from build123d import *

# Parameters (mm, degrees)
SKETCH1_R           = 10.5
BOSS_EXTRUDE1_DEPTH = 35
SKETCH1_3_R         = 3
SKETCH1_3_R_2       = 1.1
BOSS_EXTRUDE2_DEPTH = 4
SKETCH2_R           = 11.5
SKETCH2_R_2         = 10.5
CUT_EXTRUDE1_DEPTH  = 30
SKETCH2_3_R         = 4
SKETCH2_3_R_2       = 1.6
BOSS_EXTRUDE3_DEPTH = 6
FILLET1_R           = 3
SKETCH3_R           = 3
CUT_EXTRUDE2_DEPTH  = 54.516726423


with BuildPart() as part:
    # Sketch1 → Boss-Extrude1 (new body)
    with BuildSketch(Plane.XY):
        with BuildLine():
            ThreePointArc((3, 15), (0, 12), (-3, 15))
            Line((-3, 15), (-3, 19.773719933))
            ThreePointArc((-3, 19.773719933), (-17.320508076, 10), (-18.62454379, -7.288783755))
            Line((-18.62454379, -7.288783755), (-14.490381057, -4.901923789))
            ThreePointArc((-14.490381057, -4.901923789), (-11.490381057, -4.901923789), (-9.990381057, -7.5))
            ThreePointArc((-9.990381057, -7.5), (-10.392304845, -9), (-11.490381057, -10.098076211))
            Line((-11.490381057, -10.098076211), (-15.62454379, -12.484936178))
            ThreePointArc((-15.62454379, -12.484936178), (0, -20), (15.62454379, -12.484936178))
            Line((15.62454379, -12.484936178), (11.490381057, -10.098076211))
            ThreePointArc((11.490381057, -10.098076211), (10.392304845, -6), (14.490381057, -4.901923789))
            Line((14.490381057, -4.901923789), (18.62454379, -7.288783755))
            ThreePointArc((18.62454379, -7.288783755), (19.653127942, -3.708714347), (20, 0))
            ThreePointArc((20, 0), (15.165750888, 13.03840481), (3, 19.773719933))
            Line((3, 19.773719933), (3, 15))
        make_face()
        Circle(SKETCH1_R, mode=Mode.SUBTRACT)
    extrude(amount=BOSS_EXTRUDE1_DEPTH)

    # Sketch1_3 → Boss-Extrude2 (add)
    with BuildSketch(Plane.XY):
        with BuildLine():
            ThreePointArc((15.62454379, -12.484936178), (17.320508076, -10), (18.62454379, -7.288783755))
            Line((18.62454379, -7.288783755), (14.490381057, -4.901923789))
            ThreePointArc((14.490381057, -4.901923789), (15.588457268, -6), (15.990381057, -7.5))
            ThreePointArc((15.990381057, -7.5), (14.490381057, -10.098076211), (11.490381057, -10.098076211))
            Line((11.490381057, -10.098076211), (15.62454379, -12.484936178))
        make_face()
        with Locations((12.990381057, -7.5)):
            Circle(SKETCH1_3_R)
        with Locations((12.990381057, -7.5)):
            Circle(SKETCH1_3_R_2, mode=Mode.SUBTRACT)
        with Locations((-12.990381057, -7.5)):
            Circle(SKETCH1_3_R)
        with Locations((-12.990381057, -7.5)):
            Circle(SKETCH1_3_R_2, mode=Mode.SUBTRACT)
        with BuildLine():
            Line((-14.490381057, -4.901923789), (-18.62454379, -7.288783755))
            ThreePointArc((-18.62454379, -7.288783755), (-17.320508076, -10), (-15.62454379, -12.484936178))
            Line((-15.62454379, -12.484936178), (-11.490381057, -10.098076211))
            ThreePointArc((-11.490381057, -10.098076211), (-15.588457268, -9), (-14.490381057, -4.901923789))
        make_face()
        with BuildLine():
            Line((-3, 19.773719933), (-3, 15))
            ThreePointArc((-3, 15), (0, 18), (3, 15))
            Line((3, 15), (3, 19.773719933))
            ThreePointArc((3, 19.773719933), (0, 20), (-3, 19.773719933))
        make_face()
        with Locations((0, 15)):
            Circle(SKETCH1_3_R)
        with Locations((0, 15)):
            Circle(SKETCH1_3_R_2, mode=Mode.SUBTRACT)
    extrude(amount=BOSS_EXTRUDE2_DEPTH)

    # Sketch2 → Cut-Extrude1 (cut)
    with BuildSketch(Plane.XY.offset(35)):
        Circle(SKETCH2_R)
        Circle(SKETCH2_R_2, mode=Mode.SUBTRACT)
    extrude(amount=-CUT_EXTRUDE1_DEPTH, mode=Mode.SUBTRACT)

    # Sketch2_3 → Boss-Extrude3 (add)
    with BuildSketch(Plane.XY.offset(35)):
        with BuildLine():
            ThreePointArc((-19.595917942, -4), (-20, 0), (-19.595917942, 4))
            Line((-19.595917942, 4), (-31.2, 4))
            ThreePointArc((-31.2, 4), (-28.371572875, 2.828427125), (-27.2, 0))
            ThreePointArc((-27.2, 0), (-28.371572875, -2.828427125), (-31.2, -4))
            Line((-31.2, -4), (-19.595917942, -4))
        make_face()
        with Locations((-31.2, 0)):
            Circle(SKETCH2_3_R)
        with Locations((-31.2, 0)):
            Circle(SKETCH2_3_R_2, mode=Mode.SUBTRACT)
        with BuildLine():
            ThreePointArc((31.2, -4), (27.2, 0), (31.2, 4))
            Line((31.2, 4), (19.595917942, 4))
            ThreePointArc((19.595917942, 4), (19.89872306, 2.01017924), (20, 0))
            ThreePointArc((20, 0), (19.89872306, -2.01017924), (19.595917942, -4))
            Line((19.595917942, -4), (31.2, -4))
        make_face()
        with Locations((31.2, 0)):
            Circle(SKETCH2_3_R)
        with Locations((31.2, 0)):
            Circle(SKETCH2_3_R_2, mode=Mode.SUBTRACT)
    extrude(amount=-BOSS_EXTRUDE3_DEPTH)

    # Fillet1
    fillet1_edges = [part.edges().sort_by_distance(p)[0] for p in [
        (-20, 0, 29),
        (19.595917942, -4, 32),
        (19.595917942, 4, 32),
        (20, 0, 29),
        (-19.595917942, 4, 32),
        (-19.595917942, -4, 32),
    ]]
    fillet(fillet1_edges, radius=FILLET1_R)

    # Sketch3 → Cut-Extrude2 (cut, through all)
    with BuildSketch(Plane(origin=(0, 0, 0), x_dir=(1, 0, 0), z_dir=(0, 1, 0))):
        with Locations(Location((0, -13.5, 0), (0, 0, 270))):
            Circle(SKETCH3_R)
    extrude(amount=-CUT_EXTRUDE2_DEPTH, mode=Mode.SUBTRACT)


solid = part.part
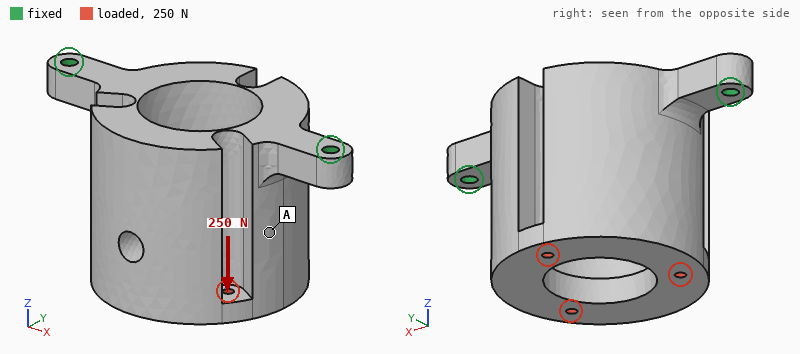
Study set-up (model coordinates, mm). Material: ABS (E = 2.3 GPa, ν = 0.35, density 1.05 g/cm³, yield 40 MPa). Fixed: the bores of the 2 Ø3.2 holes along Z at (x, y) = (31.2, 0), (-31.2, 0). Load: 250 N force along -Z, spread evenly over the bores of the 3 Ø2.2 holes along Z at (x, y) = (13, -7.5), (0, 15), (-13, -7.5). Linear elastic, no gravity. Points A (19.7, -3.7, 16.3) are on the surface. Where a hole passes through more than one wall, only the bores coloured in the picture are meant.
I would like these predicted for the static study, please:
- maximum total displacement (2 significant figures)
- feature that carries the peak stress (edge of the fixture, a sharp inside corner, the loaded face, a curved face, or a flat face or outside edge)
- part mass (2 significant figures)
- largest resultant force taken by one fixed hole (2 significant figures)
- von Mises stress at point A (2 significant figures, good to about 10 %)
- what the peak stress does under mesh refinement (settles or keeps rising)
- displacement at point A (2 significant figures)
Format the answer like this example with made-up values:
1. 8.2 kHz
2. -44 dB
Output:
1. 0.15 mm
2. edge of the fixture
3. 28 g
4. 140 N
5. 1.9 MPa
6. keeps rising
7. 0.12 mm
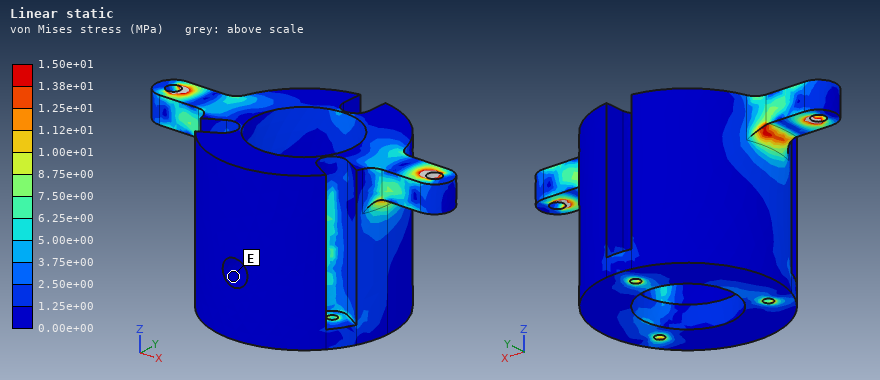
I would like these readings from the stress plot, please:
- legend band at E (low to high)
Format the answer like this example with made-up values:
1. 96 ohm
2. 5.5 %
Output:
1. 0.00e+00 to 1.25e+00 MPa
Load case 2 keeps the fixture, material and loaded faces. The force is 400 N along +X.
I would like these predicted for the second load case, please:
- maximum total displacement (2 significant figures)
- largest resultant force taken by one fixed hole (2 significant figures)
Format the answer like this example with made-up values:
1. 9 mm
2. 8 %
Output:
1. 0.41 mm
2. 310 N
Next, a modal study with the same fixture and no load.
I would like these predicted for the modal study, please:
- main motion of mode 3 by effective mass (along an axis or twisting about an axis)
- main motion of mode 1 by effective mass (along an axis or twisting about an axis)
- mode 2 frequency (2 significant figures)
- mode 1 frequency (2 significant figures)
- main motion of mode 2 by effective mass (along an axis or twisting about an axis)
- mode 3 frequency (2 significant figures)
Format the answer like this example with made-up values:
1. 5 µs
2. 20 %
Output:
1. along X
2. along Y
3. 1400 Hz
4. 310 Hz
5. along Z
6. 1500 Hz
